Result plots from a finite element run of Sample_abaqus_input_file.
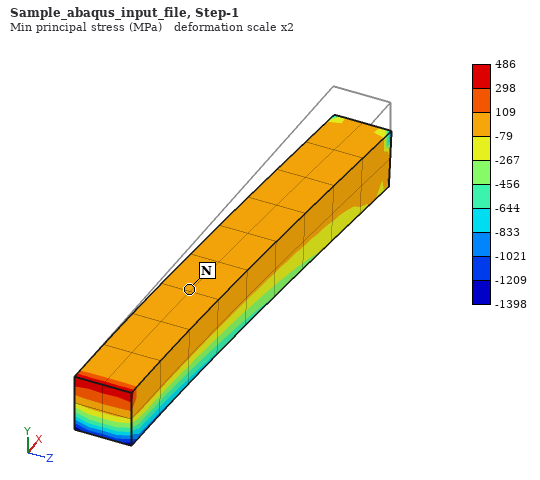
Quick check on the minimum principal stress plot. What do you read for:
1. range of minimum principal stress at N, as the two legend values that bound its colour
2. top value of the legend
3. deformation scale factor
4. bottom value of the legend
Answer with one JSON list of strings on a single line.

["-79 to 109 MPa", "486 MPa", "2", "-1398 MPa"]
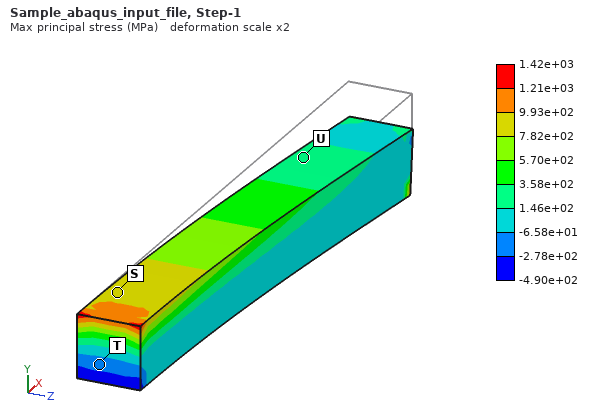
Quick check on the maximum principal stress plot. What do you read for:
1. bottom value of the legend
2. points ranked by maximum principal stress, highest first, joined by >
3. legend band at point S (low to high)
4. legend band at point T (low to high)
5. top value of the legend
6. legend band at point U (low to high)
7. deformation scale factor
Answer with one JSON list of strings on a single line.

["-4.90e+02 MPa", "S > U > T", "7.82e+02 to 9.93e+02 MPa", "-2.78e+02 to -6.58e+01 MPa", "1.42e+03 MPa", "1.46e+02 to 3.58e+02 MPa", "2"]
